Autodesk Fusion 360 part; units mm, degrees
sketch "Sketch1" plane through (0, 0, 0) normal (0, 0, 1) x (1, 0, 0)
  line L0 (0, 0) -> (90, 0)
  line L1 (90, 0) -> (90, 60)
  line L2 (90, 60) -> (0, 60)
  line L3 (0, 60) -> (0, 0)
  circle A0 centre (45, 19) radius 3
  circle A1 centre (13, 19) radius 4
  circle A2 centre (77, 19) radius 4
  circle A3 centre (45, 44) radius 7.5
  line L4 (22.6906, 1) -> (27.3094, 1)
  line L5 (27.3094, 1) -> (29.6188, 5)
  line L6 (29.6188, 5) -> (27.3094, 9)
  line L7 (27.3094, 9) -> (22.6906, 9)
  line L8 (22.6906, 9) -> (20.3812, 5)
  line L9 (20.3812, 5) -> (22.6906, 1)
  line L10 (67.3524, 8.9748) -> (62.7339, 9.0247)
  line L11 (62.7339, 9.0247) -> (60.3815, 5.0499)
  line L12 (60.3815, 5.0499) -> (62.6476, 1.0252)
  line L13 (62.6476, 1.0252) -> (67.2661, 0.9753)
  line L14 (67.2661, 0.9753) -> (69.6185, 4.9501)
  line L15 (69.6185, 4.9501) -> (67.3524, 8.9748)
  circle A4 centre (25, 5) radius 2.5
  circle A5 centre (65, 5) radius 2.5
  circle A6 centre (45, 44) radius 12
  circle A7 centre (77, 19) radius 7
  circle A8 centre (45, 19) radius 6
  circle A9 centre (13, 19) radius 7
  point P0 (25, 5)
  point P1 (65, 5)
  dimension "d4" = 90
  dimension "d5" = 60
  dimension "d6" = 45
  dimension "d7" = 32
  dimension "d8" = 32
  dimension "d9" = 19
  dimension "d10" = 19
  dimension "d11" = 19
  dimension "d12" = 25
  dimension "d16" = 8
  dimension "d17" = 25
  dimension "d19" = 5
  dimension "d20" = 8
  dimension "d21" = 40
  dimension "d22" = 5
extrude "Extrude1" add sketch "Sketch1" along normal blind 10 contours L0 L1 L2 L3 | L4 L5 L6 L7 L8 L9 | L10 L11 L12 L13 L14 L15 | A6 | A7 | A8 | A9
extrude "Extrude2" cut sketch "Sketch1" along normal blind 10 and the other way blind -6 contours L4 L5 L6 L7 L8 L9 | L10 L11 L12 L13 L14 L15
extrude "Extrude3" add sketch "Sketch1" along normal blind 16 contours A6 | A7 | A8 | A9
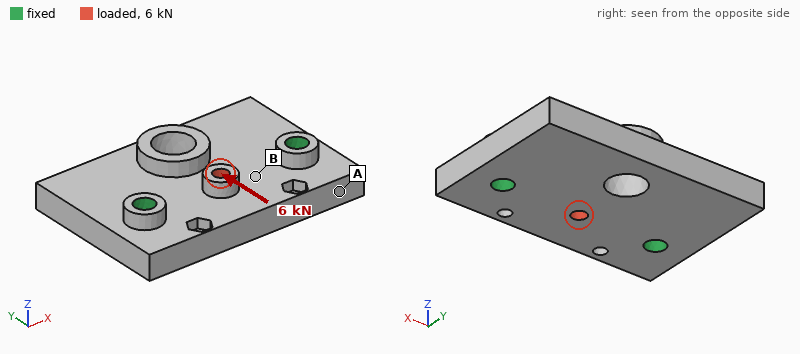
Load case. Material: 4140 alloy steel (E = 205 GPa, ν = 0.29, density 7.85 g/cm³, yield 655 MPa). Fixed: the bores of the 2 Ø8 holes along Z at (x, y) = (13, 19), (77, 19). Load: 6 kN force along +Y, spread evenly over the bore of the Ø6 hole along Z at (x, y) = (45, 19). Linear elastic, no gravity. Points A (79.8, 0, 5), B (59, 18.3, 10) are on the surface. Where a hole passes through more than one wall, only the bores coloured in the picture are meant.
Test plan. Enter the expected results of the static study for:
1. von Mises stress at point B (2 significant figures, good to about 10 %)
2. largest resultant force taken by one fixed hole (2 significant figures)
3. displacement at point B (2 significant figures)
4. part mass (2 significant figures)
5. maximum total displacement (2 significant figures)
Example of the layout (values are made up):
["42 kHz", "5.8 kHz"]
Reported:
["24 MPa", "3.0 kN", "3.2 µm", "420 g", "10 µm"]
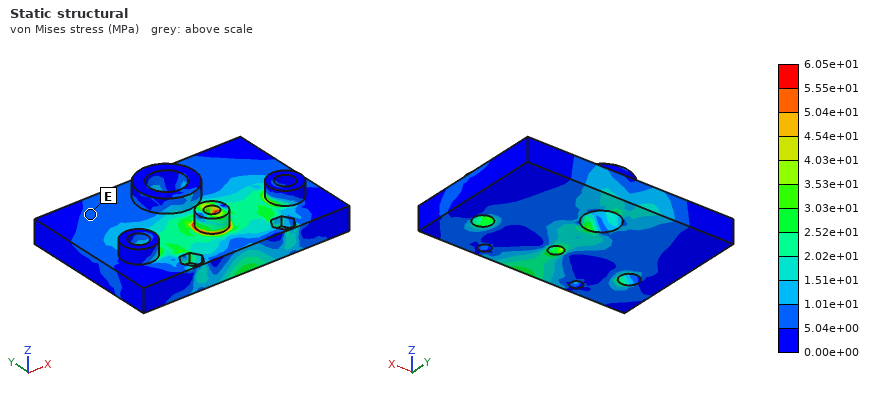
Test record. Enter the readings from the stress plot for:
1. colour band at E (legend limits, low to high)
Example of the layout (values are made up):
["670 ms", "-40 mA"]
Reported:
["5.04e+00 to 1.01e+01 MPa"]
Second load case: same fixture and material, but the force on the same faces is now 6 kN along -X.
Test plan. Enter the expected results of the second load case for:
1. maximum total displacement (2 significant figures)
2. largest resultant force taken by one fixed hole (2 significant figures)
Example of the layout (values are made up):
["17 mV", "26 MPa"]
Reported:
["6.4 µm", "3.0 kN"]
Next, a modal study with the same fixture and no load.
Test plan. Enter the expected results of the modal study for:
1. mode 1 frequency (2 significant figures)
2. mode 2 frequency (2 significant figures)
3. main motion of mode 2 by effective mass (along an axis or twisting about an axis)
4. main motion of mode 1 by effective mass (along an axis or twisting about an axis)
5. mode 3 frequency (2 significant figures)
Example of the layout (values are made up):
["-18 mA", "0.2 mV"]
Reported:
["4300 Hz", "7000 Hz", "twisting about Y", "along Z", "10 kHz"]
